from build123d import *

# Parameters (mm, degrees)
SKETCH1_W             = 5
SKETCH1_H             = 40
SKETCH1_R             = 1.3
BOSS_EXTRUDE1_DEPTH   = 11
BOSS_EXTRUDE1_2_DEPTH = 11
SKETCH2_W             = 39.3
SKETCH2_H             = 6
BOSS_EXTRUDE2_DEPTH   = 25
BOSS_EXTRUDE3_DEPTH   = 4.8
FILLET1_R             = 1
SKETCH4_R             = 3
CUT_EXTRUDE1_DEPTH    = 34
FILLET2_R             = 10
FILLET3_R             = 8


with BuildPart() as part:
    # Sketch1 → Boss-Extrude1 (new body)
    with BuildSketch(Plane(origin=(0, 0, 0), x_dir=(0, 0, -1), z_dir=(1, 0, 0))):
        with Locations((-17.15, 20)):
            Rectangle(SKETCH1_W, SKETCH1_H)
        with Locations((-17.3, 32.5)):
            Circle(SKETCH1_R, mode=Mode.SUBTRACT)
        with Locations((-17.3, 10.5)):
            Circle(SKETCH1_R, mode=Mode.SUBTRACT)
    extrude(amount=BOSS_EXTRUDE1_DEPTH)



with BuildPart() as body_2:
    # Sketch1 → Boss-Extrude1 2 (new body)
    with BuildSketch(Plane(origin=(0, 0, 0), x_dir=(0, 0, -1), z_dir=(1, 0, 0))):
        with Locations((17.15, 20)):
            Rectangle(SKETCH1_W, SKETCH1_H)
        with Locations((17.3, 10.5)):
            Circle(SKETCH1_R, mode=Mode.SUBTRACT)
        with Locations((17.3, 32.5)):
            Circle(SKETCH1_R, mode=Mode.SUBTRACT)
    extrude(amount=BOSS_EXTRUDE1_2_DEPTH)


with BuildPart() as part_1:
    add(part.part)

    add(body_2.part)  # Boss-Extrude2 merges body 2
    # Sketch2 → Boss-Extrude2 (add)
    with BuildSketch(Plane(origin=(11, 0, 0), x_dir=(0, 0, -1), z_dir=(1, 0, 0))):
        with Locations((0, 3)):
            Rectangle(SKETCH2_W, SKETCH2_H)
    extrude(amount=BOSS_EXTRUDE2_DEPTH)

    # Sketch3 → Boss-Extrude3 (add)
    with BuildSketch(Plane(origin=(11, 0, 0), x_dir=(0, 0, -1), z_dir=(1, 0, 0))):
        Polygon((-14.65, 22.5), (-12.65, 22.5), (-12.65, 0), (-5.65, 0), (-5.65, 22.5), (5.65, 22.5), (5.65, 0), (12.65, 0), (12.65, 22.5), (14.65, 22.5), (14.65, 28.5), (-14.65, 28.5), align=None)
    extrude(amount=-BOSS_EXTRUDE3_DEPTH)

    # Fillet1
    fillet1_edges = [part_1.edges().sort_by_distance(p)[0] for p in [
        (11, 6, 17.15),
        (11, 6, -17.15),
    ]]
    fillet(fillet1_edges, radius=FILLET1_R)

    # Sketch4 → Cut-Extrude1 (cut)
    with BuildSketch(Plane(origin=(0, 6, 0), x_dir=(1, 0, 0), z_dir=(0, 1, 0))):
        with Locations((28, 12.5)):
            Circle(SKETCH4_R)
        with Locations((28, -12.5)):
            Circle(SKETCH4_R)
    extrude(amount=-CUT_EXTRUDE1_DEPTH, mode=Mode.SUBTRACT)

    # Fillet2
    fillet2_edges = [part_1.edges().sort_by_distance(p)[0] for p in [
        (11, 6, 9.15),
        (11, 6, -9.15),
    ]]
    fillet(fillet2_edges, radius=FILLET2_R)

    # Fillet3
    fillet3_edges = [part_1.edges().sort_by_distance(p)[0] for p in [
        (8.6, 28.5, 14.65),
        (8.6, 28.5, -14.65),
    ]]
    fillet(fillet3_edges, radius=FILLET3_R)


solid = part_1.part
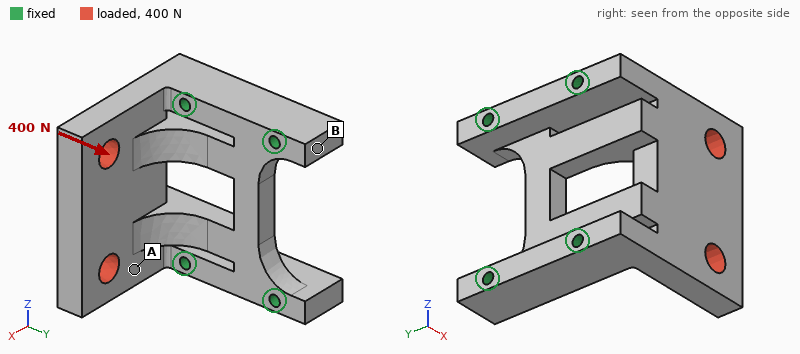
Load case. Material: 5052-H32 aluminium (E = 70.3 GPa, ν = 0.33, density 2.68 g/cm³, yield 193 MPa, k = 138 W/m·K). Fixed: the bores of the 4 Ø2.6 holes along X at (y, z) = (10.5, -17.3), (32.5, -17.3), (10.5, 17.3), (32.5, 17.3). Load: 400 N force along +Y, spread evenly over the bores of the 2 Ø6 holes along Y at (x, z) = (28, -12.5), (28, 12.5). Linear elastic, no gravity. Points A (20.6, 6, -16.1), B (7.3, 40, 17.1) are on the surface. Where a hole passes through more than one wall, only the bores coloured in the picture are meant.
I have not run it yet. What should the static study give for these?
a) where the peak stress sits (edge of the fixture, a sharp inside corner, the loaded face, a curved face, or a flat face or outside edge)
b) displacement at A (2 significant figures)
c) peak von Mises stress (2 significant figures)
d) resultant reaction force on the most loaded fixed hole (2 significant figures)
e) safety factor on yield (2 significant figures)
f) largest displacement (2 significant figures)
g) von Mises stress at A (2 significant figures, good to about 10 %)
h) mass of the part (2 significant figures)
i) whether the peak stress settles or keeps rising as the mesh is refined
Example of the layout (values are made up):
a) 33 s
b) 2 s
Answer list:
a) a curved face
b) 20 µm
c) 120 MPa
d) 150 N
e) 1.5
f) 57 µm
g) 13 MPa
h) 34 g
i) settles
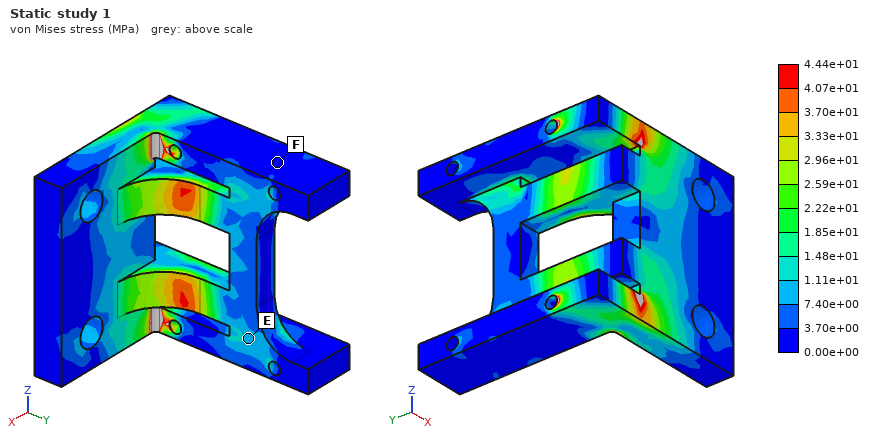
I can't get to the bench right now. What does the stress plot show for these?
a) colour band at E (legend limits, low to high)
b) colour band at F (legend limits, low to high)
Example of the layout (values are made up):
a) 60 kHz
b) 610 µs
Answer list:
a) 7.40e+00 to 1.11e+01 MPa
b) 0.00e+00 to 3.70e+00 MPa
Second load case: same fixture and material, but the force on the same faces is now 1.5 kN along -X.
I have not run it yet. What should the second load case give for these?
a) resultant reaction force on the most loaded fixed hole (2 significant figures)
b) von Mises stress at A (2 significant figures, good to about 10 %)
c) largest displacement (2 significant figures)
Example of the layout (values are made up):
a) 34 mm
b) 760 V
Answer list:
a) 780 N
b) 12 MPa
c) 24 µm
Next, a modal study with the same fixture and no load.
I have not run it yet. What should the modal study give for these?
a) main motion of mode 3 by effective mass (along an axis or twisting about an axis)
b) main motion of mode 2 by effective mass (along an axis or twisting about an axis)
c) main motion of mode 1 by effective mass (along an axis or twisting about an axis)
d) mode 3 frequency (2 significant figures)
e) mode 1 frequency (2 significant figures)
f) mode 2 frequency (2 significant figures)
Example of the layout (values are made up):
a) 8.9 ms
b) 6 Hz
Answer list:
a) along Z
b) along Z
c) along Y
d) 11 kHz
e) 4900 Hz
f) 9900 Hz
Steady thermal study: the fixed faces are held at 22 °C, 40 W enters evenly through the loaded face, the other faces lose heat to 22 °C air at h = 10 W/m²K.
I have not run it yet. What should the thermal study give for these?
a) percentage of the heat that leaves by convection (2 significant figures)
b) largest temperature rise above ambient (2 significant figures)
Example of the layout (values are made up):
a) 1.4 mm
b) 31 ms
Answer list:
a) 3.3 %
b) 52 K
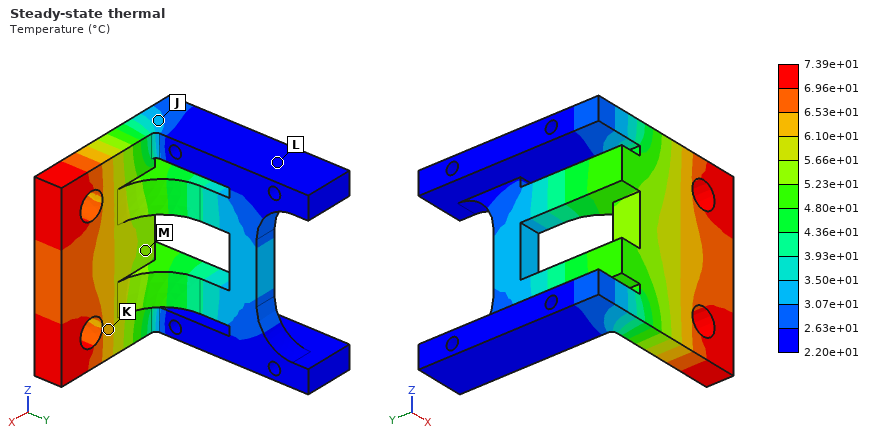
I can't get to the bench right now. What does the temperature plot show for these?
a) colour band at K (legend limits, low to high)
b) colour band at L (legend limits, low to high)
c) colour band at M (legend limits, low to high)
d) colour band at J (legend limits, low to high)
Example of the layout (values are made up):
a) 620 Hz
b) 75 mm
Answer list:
a) 6.10e+01 to 6.53e+01 °C
b) 2.20e+01 to 2.63e+01 °C
c) 5.23e+01 to 5.66e+01 °C
d) 3.07e+01 to 3.50e+01 °C
